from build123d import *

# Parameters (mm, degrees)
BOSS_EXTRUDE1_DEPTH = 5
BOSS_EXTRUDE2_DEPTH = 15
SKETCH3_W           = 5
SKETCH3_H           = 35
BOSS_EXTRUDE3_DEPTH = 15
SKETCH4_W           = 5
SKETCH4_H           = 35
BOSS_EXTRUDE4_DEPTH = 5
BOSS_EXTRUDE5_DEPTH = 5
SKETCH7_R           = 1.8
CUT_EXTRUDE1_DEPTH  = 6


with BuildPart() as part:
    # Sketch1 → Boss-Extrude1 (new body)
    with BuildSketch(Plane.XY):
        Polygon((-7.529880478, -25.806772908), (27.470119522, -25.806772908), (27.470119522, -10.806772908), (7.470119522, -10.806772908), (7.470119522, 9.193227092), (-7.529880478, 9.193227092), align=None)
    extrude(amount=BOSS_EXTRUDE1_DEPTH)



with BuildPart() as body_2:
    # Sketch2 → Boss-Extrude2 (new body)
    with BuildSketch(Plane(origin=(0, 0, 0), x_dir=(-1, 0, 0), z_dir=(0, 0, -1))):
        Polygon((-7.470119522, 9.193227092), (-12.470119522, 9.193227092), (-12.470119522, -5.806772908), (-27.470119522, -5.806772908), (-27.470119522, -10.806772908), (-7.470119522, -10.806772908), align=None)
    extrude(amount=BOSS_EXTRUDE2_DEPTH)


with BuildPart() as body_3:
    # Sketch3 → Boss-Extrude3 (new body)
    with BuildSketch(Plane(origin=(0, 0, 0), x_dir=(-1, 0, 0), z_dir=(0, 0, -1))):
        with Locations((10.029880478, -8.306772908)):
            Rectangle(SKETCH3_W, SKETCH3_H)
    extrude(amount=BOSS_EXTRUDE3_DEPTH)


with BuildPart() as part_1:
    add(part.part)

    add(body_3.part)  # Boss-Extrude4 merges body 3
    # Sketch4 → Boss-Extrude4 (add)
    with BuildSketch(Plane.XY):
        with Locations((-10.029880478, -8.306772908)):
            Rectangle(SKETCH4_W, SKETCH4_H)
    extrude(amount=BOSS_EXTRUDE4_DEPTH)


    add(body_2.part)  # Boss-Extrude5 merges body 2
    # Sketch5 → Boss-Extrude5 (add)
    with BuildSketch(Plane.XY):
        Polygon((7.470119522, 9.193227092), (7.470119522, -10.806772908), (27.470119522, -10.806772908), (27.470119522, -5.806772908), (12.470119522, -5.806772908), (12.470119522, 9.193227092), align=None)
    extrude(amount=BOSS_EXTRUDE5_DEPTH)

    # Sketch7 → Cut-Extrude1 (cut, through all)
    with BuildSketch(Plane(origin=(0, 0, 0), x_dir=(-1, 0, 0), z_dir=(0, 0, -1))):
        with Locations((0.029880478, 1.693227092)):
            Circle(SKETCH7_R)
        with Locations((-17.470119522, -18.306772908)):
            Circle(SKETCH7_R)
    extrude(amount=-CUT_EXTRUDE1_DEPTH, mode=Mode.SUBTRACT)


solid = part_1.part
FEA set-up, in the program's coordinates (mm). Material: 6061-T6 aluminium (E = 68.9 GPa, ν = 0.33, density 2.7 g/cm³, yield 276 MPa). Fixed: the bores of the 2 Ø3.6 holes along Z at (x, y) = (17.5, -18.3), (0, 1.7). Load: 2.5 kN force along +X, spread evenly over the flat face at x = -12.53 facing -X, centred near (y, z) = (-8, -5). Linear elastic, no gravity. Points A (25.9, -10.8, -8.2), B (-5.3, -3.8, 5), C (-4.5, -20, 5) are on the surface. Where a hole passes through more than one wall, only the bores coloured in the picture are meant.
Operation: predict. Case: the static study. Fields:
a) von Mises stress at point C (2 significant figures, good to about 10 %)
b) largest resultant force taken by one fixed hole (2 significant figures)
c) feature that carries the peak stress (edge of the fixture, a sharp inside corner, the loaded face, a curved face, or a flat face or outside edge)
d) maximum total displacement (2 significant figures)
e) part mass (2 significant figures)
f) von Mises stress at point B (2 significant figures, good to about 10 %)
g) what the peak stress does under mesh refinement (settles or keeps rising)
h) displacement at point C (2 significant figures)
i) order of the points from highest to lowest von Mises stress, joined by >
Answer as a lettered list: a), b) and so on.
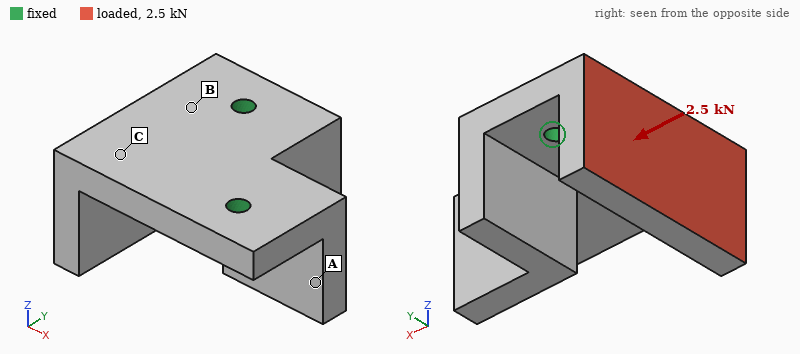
a) 78 MPa
b) 1.3 kN
c) edge of the fixture
d) 0.26 mm
e) 30 g
f) 110 MPa
g) keeps rising
h) 0.053 mm
i) B > C > A
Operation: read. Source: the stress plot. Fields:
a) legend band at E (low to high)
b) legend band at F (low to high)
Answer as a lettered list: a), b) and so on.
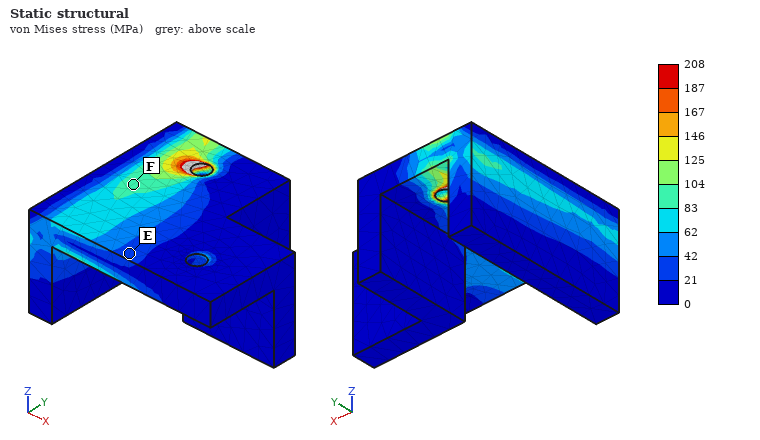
a) 21 to 42 MPa
b) 83 to 104 MPa
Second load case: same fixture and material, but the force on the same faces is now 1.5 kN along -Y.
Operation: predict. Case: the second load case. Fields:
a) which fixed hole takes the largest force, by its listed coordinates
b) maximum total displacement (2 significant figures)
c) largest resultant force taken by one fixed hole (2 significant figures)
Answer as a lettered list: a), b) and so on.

a) (0, 1.7)
b) 99 µm
c) 1.7 kN
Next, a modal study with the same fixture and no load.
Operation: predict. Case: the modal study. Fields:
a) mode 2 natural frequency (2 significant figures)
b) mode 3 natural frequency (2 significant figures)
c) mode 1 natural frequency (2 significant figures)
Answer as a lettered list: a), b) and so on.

a) 7800 Hz
b) 9300 Hz
c) 4600 Hz
